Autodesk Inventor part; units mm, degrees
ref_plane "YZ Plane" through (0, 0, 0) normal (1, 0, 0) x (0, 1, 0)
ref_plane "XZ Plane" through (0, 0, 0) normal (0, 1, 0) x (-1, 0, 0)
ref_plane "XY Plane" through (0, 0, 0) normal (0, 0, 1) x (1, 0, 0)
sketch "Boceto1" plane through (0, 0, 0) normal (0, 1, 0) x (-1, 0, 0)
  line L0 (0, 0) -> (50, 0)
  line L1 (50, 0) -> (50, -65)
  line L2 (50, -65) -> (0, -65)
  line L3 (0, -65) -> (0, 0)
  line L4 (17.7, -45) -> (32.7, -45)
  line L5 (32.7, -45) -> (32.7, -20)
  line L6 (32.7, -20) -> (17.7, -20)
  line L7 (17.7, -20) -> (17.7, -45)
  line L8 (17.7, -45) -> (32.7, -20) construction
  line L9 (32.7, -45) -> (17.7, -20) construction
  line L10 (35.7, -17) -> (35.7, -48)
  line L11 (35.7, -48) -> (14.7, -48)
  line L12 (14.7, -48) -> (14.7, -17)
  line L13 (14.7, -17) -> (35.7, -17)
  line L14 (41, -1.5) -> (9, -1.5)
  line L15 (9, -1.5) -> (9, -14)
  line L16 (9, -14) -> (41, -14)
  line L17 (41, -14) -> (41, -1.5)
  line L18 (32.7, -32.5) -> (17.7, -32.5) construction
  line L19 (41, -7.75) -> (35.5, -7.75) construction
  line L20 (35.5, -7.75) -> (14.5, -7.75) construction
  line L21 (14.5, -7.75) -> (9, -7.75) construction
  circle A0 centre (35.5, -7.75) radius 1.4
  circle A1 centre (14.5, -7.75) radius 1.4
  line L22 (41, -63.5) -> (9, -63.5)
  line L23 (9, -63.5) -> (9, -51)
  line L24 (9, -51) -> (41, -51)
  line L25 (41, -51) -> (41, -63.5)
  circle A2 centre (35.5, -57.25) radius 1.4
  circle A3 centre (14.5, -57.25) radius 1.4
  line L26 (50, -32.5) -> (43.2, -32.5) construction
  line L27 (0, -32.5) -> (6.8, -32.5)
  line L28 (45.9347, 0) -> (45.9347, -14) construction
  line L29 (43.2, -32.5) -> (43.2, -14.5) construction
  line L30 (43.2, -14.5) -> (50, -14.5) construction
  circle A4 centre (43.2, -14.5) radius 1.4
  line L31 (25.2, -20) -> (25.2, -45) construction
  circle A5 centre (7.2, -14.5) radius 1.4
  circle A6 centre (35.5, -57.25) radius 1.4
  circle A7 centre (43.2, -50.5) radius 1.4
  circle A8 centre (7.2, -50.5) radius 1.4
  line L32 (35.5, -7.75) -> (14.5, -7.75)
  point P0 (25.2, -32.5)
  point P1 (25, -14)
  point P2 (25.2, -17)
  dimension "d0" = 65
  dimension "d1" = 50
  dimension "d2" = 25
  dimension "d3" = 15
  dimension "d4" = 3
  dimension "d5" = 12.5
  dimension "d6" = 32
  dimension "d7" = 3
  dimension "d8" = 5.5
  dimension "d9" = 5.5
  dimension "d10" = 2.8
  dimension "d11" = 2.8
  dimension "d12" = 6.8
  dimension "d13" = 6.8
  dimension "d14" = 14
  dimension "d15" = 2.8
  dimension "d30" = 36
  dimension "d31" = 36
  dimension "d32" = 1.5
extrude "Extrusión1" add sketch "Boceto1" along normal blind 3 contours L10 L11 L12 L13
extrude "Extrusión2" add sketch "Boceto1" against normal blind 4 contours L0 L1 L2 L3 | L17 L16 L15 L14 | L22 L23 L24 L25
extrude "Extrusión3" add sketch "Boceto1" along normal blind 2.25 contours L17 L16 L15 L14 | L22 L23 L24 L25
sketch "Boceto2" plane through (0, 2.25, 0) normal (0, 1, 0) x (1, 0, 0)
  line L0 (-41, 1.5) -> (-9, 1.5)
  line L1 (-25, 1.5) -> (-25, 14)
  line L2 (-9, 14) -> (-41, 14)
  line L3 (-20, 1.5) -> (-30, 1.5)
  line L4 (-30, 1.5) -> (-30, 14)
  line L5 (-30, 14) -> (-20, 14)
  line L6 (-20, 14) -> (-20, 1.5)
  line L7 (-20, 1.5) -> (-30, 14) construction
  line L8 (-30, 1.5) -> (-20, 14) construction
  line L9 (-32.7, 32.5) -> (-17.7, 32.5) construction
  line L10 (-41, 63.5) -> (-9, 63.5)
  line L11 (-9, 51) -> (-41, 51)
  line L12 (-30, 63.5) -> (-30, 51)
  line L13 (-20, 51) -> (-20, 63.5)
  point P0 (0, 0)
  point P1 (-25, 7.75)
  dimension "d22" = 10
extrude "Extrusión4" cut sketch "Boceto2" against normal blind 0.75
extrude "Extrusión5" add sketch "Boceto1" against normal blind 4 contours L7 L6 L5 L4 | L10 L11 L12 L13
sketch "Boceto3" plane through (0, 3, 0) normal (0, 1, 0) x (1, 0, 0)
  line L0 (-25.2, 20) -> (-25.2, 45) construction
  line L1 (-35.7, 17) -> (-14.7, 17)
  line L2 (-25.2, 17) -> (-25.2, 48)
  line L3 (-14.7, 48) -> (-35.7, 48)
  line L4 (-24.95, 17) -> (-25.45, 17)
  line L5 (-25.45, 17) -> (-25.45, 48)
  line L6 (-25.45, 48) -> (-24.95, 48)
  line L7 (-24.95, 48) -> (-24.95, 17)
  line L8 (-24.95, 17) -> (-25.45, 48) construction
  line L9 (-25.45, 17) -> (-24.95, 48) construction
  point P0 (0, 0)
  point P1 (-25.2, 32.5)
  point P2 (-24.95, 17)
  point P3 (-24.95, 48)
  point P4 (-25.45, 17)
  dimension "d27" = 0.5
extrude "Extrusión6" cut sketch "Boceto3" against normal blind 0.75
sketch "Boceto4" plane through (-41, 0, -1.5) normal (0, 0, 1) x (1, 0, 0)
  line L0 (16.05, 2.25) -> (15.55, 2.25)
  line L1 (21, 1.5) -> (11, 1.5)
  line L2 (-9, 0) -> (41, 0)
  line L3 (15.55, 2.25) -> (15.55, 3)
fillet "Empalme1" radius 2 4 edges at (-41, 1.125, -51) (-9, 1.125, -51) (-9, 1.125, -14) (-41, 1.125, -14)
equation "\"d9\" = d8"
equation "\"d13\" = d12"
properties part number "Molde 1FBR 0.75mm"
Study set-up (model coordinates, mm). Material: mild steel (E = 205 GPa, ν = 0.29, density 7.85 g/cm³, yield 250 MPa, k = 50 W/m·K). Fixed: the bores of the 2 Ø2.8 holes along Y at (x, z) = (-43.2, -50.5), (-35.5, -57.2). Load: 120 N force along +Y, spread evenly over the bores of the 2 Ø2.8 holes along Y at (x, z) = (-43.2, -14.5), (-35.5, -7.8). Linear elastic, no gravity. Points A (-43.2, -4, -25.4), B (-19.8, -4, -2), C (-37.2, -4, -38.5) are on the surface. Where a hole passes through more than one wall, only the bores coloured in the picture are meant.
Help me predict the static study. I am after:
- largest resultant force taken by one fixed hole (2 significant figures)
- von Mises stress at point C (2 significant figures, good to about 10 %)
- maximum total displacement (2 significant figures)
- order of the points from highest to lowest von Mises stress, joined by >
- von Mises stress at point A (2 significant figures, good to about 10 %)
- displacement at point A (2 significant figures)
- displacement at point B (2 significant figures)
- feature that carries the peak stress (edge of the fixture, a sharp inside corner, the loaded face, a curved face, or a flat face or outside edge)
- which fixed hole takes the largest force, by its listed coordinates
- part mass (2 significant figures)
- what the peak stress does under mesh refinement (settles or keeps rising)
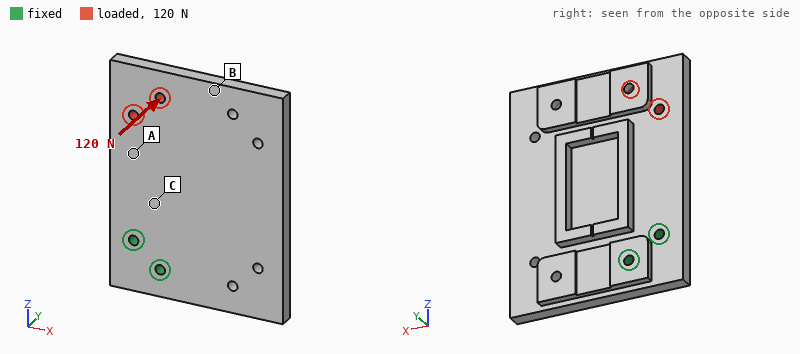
210 N
21 MPa
73 µm
C > A > B
12 MPa
29 µm
64 µm
edge of the fixture
(-43.2, -50.5)
120 g
keeps rising
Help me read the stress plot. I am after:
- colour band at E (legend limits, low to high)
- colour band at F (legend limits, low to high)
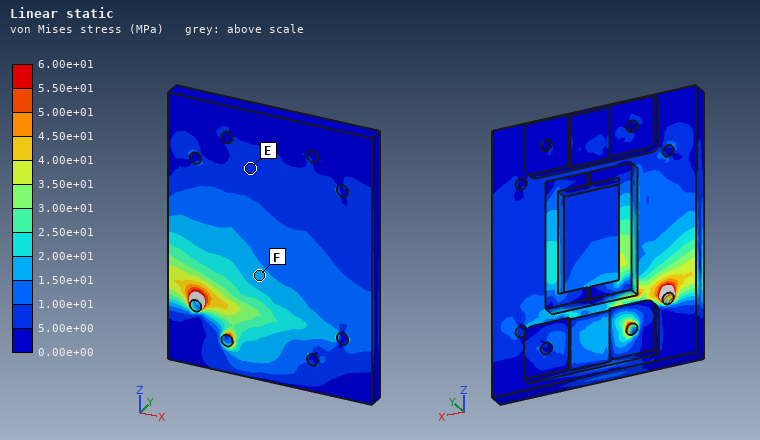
5.00e+00 to 1.00e+01 MPa
1.50e+01 to 2.00e+01 MPa
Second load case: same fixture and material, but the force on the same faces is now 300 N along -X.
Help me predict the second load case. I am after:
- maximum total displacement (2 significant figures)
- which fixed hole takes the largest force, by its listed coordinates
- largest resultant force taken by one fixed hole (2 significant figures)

14 µm
(-43.2, -50.5)
1.1 kN
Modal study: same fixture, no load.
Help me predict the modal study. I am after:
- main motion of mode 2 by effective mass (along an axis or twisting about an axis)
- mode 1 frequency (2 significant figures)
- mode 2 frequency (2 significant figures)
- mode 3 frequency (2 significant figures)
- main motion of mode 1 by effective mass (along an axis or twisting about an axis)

twisting about Z
990 Hz
2400 Hz
3400 Hz
along Y
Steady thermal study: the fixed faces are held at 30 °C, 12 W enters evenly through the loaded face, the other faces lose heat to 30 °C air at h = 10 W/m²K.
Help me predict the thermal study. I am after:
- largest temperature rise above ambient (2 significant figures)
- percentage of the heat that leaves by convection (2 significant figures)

63 K
20 %
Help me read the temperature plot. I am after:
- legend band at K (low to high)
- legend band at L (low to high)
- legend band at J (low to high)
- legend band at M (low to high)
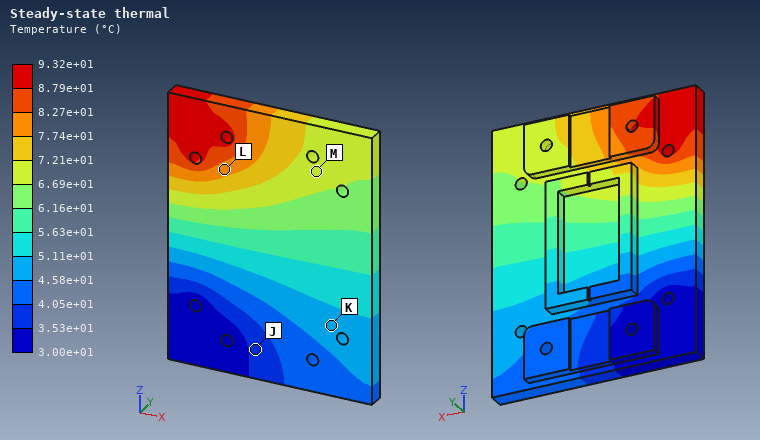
4.58e+01 to 5.11e+01 °C
7.74e+01 to 8.27e+01 °C
3.53e+01 to 4.05e+01 °C
6.69e+01 to 7.21e+01 °C
